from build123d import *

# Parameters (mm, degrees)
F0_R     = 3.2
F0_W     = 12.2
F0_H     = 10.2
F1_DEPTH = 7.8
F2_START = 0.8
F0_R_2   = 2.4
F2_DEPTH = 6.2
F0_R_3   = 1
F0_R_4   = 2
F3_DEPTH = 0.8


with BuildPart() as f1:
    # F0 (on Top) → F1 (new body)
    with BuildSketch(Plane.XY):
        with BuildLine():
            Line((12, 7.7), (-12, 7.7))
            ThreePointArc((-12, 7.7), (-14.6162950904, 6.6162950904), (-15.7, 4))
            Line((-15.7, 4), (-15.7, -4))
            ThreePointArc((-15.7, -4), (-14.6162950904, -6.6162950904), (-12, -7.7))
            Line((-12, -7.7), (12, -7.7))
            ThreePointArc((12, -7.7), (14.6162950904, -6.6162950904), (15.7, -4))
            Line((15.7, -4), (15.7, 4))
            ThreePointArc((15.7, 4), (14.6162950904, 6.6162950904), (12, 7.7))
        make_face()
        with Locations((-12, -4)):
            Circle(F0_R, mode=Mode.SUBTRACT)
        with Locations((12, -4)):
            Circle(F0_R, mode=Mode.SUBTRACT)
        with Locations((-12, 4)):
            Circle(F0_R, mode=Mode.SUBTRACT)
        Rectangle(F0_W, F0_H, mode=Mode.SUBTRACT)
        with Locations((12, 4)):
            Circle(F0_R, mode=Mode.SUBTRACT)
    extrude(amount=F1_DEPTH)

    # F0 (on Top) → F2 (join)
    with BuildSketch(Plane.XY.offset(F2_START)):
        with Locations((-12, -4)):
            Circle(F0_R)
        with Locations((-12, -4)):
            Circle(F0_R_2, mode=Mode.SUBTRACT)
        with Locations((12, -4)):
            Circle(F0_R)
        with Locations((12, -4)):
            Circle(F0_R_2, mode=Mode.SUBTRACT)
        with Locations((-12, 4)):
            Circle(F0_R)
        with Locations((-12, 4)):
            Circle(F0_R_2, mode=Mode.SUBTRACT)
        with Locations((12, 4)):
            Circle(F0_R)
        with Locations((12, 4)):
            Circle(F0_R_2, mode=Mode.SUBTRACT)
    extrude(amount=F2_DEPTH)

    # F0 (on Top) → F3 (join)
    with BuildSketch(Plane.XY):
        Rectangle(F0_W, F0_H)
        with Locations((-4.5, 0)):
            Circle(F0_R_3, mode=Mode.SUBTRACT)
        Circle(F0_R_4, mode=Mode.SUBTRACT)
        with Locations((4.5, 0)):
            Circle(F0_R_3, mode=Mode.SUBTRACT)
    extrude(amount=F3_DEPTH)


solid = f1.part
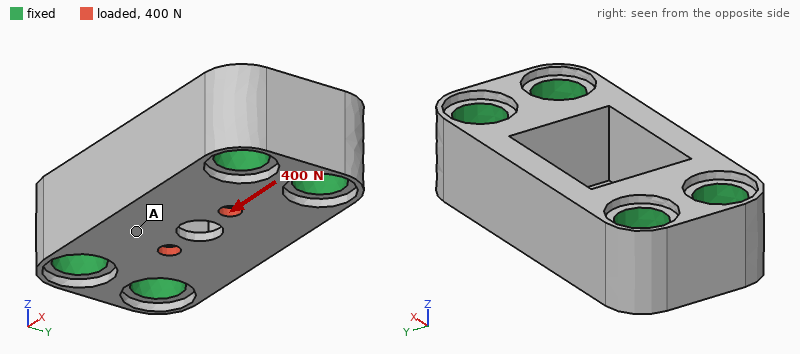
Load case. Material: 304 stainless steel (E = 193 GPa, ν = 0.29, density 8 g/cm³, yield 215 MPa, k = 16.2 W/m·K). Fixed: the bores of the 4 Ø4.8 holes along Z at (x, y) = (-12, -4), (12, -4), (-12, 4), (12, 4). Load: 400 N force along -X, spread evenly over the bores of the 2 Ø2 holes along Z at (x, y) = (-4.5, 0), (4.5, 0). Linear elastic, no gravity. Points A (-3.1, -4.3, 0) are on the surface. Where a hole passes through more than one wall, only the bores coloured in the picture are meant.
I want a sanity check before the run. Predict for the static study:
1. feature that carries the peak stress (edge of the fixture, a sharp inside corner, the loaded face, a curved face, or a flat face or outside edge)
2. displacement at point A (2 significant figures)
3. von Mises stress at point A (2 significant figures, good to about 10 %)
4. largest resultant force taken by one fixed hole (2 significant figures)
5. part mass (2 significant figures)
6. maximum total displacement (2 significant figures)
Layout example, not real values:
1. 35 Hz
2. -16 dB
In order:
1. the loaded face
2. 0.19 µm
3. 5.6 MPa
4. 110 N
5. 17 g
6. 1.2 µm
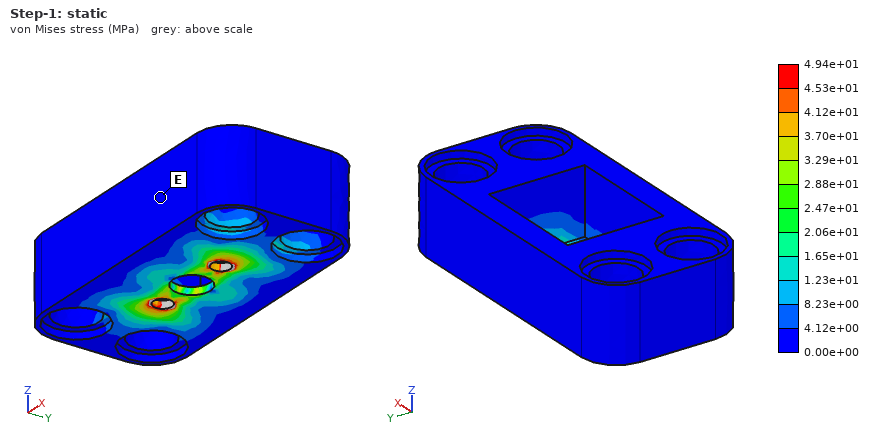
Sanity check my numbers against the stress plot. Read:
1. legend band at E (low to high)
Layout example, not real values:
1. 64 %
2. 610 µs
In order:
1. 0.00e+00 to 4.12e+00 MPa
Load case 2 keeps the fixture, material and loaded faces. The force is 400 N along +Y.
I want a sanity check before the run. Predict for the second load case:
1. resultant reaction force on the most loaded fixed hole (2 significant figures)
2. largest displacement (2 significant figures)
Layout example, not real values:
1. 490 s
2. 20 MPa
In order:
1. 130 N
2. 1.2 µm
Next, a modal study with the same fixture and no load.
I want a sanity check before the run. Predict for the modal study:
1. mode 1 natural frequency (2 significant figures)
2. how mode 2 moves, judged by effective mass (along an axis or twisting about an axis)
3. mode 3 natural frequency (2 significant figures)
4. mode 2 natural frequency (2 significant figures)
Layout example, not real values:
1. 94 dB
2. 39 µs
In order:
1. 48 kHz
2. along Y
3. 56 kHz
4. 53 kHz
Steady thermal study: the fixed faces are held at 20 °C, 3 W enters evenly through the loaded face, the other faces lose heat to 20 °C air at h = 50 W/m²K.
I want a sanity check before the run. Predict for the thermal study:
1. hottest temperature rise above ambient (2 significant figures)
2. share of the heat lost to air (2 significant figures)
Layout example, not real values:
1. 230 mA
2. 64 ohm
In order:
1. 41 K
2. 11 %
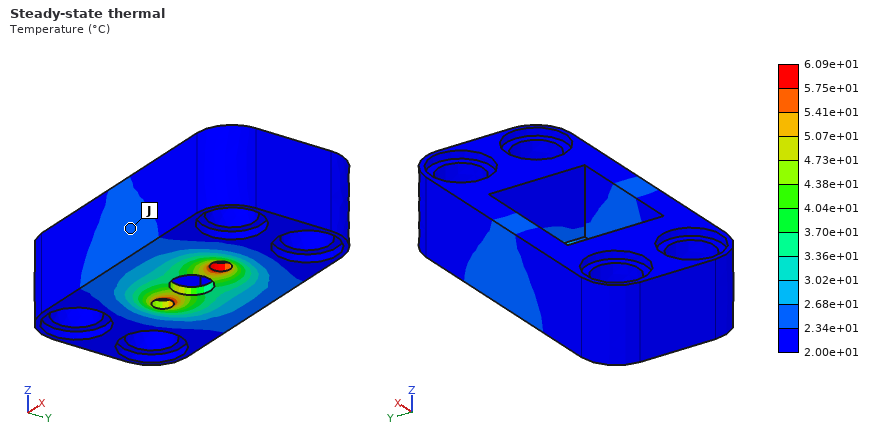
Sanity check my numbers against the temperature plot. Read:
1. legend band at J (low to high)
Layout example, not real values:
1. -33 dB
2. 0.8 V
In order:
1. 2.34e+01 to 2.68e+01 °C
